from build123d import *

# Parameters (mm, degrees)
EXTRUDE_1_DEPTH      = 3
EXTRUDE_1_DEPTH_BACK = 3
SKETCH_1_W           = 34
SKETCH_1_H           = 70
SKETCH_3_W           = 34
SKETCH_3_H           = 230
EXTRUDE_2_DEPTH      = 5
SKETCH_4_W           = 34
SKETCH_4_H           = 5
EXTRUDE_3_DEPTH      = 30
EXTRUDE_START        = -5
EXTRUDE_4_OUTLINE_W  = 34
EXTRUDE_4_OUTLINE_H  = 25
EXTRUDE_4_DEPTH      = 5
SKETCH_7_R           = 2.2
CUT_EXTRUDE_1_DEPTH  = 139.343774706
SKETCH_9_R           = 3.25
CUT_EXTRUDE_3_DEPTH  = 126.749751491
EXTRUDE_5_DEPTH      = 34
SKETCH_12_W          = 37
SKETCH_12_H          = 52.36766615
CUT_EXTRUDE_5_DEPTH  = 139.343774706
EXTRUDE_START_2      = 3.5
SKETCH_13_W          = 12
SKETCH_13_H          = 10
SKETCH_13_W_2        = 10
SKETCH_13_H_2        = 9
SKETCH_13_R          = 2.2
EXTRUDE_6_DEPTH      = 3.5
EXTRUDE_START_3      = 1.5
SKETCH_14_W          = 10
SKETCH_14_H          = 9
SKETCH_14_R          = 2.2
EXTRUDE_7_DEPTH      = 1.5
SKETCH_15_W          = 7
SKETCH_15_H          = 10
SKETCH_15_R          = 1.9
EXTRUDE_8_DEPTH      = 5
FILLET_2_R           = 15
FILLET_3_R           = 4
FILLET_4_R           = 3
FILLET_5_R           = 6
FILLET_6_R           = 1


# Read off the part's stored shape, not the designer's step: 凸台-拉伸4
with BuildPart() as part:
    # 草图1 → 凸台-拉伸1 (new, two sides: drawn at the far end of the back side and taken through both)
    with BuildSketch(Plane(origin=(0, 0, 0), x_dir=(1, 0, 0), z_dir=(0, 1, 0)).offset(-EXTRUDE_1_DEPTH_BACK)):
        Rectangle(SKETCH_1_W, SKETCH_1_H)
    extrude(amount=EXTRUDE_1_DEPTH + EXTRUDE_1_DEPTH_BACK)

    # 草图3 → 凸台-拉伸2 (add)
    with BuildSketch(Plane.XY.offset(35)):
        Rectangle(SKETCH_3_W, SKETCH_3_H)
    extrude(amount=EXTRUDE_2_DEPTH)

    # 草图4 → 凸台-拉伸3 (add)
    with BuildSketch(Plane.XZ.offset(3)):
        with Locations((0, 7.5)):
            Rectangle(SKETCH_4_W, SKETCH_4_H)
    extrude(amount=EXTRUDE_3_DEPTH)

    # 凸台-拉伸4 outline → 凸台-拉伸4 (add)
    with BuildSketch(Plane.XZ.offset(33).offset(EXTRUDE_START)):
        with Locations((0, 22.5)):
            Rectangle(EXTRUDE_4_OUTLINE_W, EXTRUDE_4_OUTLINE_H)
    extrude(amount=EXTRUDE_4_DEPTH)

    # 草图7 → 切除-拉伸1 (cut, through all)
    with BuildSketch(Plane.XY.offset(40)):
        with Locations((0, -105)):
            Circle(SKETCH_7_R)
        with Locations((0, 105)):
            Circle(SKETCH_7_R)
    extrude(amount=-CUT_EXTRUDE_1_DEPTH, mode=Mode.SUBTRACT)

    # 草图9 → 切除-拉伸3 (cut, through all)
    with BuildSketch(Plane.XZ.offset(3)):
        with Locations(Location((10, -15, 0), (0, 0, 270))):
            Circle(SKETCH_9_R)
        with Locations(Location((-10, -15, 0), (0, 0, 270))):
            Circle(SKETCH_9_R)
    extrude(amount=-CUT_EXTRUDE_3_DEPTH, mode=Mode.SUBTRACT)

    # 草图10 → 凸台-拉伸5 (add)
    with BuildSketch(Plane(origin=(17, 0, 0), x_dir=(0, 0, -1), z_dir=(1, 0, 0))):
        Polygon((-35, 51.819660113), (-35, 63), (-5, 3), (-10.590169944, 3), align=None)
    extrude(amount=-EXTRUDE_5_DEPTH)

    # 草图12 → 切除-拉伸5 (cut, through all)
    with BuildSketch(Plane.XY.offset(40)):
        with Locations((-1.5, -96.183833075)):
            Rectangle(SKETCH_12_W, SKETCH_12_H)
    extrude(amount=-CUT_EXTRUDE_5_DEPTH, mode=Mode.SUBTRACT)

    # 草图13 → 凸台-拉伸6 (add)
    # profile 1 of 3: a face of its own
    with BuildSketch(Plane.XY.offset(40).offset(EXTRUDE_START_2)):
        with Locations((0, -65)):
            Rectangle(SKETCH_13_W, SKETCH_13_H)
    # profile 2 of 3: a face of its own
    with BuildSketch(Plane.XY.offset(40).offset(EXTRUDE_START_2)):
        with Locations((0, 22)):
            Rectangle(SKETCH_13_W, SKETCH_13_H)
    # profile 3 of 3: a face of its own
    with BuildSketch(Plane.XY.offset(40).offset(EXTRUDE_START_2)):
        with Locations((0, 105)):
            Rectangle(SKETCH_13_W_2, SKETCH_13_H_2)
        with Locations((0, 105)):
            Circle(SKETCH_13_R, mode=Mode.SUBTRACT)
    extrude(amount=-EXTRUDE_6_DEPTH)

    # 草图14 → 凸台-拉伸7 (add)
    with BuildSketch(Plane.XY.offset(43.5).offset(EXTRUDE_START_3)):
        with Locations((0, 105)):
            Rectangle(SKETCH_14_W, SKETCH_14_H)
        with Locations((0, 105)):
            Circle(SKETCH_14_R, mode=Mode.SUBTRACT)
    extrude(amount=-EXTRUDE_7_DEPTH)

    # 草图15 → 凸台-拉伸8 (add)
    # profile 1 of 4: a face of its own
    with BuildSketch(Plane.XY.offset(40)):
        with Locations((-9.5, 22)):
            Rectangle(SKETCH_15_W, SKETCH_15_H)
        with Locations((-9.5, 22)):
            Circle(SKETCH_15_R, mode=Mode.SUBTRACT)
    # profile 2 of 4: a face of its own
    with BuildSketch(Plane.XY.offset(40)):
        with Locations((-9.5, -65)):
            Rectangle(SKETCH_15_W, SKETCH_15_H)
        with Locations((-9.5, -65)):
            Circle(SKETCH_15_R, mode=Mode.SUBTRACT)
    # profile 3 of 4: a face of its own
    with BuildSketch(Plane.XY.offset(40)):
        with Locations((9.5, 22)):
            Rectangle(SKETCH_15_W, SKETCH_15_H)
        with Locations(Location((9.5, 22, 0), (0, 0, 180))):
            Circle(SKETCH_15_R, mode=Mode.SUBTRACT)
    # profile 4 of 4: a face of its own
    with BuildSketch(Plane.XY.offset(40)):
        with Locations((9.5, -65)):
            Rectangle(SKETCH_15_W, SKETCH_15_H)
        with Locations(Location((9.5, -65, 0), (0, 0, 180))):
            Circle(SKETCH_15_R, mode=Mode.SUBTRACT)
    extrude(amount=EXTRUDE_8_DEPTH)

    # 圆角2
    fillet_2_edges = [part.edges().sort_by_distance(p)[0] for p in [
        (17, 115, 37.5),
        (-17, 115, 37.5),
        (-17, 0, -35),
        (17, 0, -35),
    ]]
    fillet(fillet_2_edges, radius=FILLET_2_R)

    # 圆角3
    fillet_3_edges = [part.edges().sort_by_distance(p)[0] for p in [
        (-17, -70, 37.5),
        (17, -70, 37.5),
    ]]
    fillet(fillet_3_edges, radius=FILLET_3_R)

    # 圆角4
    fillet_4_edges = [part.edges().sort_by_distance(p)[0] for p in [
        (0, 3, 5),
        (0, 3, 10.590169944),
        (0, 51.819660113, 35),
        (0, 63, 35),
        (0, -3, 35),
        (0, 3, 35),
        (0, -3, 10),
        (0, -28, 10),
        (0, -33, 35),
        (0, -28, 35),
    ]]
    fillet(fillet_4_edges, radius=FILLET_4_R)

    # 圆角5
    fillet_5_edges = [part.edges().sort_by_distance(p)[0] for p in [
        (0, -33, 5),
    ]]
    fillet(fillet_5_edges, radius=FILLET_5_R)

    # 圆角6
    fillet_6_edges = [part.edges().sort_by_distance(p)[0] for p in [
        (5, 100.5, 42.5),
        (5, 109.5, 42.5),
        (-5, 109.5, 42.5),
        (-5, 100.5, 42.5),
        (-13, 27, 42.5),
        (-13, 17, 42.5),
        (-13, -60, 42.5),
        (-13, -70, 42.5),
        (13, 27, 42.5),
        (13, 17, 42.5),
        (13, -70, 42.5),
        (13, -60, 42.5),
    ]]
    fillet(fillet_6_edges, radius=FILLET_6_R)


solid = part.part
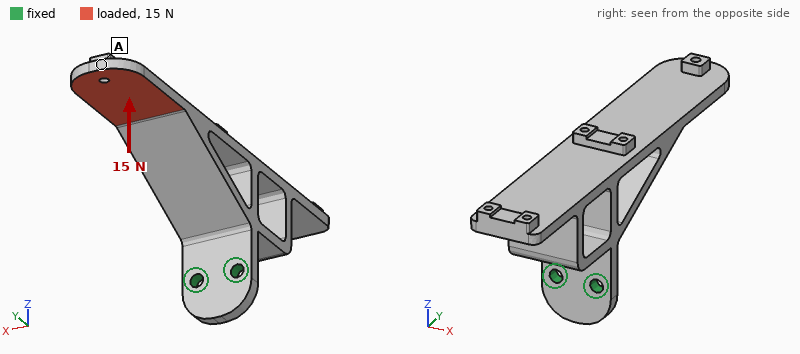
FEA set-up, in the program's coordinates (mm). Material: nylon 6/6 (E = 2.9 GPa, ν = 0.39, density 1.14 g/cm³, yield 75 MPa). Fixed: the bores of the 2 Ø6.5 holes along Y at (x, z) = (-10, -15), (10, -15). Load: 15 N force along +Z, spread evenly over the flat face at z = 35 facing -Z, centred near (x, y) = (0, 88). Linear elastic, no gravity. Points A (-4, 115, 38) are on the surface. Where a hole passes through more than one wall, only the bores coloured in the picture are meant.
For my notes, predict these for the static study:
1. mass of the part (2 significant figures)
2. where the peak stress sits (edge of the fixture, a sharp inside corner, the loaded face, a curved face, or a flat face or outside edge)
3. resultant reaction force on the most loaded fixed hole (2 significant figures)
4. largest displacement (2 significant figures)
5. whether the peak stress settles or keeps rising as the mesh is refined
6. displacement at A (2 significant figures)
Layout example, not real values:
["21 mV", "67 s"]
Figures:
["77 g", "edge of the fixture", "7.8 N", "2.3 mm", "keeps rising", "2.3 mm"]
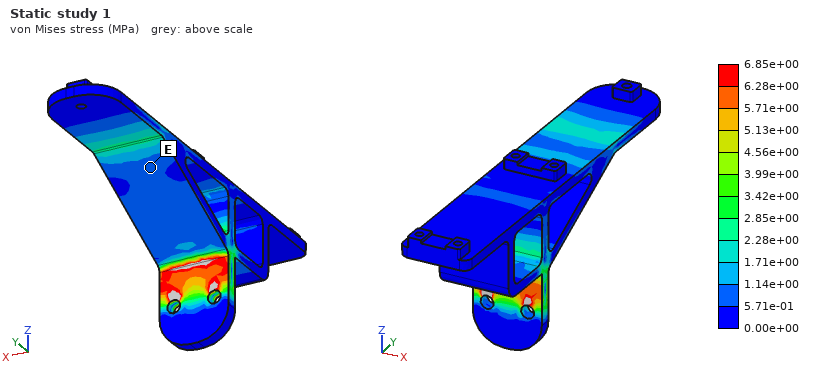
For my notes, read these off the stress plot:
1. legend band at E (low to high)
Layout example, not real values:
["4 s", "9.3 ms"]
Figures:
["5.71e-01 to 1.14e+00 MPa"]
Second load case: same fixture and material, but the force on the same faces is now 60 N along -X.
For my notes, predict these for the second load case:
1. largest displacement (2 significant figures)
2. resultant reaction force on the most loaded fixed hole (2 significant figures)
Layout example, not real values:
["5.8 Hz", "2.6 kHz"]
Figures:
["2.4 mm", "250 N"]
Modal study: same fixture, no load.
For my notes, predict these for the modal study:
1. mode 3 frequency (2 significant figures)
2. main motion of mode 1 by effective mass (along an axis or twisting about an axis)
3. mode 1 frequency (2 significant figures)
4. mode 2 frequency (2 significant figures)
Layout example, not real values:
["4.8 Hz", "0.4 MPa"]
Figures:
["430 Hz", "along Y", "97 Hz", "210 Hz"]
